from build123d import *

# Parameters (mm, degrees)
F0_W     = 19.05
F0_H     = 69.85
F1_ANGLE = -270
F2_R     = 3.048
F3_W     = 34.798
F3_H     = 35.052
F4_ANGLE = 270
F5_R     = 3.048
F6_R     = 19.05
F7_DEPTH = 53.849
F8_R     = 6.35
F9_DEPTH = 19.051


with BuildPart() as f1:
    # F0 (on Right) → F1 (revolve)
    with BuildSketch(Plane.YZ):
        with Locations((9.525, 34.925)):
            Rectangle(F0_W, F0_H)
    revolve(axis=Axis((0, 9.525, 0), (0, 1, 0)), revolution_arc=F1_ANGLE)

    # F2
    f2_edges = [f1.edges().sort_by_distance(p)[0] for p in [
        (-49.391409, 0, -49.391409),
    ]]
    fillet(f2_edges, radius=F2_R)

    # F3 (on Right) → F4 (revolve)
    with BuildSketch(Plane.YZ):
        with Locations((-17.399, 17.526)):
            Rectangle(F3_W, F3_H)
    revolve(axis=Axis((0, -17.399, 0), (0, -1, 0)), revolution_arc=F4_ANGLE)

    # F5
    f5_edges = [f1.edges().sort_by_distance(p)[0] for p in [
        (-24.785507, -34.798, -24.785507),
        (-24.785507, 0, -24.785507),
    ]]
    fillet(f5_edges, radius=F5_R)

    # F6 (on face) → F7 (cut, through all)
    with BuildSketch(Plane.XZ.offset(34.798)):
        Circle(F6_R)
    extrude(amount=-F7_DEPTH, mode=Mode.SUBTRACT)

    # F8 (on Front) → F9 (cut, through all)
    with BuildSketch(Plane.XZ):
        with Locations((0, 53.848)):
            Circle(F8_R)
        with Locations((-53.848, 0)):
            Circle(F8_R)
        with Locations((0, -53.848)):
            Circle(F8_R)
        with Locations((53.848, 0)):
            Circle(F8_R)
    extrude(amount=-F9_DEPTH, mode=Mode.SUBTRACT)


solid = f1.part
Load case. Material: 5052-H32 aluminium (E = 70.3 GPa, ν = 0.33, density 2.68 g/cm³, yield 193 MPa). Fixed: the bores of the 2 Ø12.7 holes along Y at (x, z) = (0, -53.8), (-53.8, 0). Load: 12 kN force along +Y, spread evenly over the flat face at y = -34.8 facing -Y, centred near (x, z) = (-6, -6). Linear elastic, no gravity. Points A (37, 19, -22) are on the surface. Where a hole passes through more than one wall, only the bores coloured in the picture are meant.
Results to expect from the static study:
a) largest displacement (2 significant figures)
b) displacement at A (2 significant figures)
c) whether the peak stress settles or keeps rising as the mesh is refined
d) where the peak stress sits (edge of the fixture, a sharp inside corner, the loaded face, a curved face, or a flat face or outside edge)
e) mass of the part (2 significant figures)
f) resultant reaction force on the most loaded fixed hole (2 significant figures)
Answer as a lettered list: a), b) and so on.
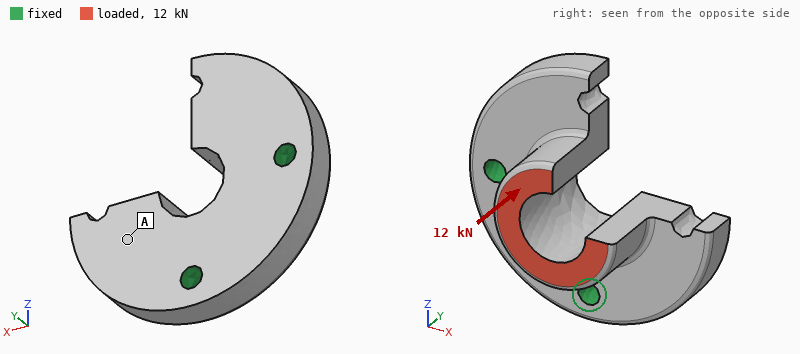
a) 0.11 mm
b) 0.061 mm
c) keeps rising
d) edge of the fixture
e) 710 g
f) 6.1 kN
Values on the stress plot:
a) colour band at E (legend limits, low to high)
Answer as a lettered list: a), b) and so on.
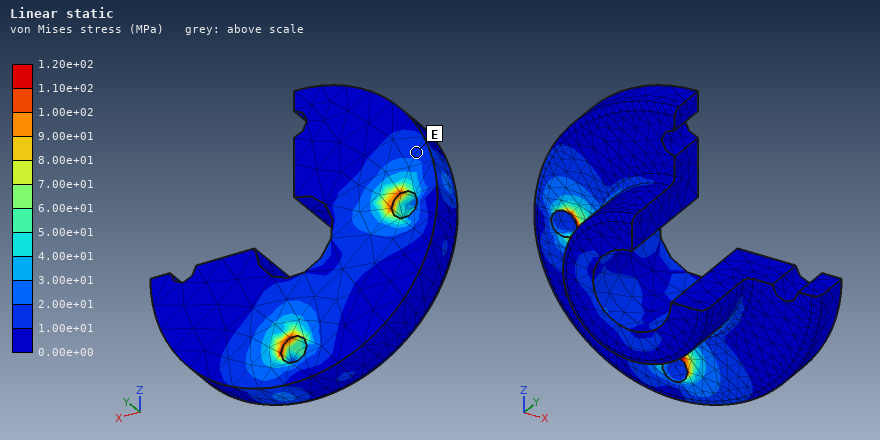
a) 1.00e+01 to 2.00e+01 MPa
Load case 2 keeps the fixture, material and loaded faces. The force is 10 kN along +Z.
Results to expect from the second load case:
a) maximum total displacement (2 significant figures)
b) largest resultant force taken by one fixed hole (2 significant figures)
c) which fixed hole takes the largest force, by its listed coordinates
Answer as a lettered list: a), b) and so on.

a) 0.15 mm
b) 8.0 kN
c) (0, -53.8)
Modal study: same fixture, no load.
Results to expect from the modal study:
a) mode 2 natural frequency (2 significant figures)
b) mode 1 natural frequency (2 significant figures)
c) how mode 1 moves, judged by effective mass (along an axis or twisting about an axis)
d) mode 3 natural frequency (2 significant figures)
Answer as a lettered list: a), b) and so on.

a) 3400 Hz
b) 2500 Hz
c) along Y
d) 4900 Hz
